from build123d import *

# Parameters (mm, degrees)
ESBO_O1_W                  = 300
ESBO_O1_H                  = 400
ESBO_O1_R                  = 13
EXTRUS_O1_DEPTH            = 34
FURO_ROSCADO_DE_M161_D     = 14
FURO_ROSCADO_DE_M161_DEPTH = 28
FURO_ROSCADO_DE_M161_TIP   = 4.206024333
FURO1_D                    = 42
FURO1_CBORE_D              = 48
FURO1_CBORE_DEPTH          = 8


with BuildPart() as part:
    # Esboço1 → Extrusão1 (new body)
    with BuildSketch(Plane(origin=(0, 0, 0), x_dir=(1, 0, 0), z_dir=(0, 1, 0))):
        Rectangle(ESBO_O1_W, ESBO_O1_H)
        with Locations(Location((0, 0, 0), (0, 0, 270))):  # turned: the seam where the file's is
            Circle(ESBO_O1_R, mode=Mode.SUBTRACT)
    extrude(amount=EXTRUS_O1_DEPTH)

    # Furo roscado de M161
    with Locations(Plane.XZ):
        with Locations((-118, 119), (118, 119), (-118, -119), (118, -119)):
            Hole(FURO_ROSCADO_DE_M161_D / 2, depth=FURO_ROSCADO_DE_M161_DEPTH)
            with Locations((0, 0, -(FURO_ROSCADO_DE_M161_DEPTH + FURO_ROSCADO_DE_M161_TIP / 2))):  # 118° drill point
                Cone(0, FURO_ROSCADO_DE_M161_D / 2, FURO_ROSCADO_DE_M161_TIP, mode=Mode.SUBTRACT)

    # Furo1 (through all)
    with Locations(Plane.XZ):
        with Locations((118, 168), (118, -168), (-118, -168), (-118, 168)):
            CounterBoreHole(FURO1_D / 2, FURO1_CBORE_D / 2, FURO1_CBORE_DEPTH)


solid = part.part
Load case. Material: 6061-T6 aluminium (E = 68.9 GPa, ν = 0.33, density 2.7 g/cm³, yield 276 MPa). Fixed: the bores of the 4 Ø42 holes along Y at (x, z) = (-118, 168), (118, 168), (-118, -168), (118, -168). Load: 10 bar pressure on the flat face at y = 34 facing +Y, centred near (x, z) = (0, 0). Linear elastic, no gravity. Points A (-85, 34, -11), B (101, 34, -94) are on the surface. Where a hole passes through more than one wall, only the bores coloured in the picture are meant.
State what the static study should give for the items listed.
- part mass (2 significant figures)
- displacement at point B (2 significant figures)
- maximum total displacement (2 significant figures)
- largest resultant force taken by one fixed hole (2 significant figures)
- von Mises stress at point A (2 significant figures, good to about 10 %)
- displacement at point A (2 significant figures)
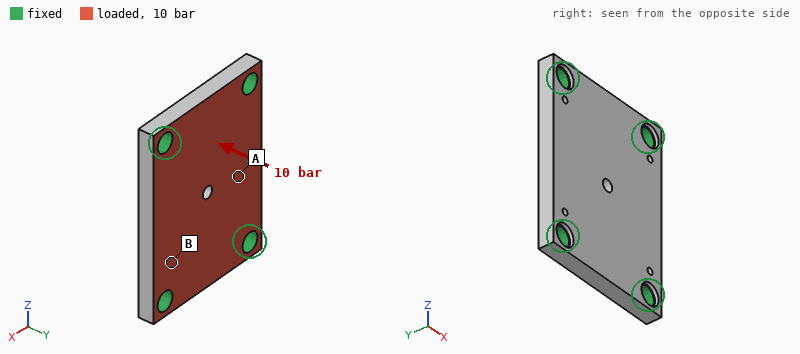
10 kg
0.10 mm
0.22 mm
29 kN
24 MPa
0.20 mm
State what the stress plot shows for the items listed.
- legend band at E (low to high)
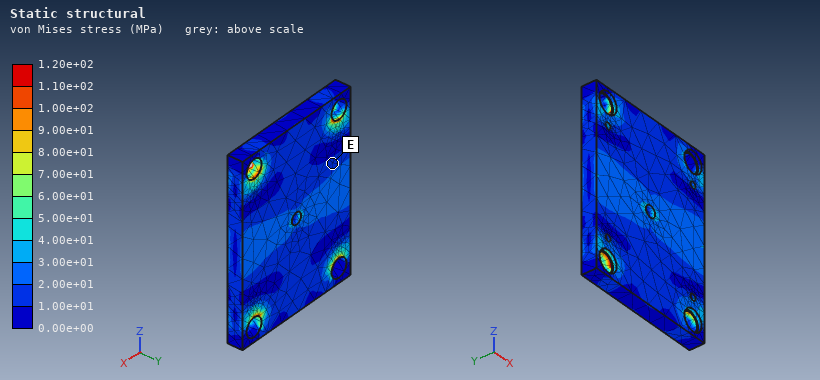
1.00e+01 to 2.00e+01 MPa
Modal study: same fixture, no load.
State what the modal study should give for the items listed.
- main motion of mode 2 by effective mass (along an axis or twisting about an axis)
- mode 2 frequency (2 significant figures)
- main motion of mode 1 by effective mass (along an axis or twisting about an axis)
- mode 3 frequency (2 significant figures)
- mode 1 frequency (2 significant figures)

twisting about Z
1900 Hz
along Y
2800 Hz
1300 Hz
